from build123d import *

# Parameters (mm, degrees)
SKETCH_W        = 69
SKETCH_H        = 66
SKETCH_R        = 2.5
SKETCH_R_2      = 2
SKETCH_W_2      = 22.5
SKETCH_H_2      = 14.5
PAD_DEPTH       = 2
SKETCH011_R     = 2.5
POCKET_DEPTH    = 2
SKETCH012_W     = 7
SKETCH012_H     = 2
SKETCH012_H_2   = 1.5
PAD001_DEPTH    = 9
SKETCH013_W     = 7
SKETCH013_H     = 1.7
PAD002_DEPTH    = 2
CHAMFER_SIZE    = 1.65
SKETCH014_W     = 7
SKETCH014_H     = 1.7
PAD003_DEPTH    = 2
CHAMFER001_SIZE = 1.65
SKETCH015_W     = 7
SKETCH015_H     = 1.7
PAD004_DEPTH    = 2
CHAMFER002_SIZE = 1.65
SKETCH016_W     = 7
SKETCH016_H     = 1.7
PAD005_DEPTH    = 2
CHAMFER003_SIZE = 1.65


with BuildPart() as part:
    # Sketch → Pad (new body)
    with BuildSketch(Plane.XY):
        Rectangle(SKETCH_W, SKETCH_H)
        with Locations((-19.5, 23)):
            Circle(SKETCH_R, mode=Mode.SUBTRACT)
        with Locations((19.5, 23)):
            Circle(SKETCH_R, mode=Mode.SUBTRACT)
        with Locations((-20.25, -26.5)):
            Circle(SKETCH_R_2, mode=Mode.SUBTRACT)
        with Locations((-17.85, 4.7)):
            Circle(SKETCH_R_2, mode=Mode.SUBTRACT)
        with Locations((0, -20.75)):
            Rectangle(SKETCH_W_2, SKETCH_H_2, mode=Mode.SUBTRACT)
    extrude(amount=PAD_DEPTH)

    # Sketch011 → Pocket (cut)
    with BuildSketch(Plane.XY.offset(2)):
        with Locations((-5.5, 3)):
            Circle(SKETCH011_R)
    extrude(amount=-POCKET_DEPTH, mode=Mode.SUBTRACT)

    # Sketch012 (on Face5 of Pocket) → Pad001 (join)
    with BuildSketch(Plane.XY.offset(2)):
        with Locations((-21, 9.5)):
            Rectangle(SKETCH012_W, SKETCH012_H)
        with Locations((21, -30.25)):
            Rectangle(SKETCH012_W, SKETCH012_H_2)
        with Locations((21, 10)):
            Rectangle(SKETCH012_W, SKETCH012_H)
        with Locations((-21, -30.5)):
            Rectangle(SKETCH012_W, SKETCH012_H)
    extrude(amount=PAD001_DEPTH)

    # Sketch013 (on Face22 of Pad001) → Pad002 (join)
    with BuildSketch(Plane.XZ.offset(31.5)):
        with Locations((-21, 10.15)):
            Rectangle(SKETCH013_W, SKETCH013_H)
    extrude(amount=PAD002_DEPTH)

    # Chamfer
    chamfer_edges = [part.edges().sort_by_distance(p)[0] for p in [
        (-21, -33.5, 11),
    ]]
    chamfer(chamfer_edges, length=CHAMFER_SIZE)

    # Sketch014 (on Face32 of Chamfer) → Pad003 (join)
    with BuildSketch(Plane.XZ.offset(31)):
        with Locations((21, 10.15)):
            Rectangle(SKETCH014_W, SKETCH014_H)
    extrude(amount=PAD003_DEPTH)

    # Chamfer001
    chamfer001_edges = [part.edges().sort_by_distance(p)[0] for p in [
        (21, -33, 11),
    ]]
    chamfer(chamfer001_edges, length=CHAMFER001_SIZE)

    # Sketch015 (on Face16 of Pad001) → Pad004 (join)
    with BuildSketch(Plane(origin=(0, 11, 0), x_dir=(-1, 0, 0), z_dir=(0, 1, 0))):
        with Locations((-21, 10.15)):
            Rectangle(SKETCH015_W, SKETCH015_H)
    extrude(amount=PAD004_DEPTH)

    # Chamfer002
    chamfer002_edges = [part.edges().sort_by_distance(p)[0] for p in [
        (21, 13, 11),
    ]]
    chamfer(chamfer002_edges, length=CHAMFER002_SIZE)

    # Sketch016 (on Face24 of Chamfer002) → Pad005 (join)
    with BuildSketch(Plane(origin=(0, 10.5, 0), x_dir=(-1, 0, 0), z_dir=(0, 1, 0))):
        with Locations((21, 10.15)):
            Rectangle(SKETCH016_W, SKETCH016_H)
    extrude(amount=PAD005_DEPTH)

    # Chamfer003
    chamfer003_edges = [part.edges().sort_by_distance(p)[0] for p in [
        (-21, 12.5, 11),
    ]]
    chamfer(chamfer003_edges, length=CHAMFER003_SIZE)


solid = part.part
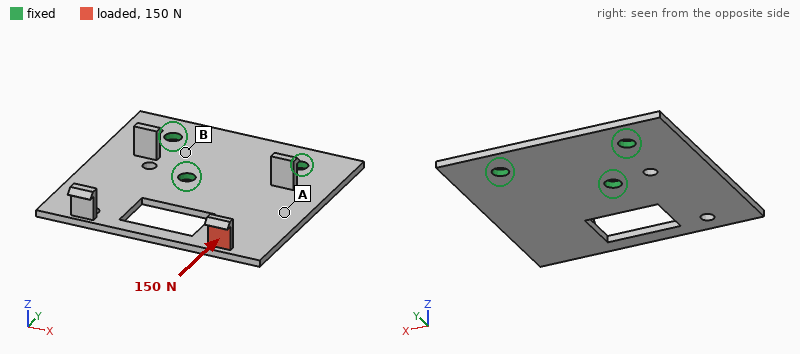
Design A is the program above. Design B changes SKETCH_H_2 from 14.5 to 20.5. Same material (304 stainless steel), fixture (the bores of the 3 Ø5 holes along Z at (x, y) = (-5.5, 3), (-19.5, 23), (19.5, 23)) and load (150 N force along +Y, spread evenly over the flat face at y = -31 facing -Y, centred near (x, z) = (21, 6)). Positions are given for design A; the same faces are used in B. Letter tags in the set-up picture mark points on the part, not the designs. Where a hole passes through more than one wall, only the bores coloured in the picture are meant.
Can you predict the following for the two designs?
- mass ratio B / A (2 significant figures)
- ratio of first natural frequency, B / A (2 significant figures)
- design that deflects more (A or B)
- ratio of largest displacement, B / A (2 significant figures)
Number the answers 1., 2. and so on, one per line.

1. 0.97
2. 0.97
3. B
4. 1.1
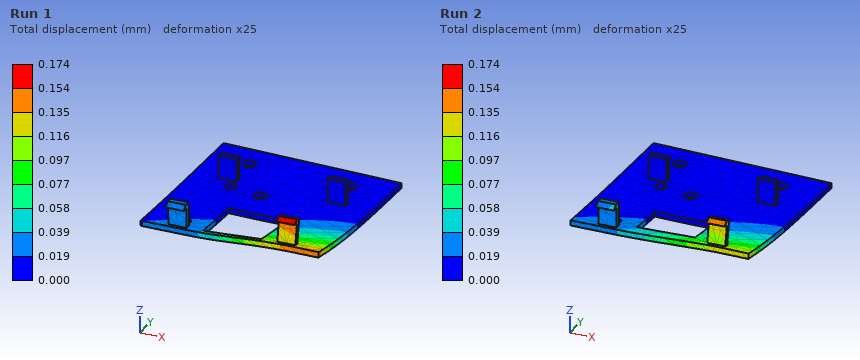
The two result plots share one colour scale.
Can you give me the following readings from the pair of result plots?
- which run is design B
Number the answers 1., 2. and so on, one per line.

1. Run 1
